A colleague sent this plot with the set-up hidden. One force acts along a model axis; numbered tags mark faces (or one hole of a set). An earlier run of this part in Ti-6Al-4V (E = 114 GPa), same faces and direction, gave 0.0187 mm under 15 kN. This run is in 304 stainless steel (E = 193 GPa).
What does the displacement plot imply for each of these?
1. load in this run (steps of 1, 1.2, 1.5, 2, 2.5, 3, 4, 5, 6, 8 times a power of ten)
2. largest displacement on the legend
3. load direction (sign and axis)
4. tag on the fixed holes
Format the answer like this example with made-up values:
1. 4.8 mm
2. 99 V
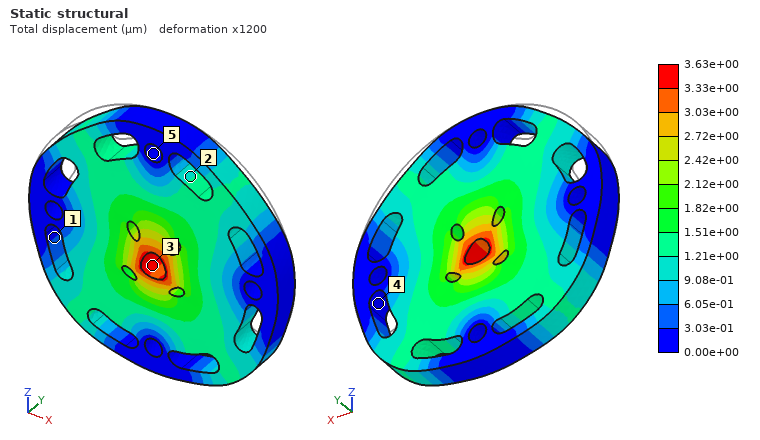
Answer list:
1. 5 kN
2. 3.63e+00 µm
3. -Z
4. 5
